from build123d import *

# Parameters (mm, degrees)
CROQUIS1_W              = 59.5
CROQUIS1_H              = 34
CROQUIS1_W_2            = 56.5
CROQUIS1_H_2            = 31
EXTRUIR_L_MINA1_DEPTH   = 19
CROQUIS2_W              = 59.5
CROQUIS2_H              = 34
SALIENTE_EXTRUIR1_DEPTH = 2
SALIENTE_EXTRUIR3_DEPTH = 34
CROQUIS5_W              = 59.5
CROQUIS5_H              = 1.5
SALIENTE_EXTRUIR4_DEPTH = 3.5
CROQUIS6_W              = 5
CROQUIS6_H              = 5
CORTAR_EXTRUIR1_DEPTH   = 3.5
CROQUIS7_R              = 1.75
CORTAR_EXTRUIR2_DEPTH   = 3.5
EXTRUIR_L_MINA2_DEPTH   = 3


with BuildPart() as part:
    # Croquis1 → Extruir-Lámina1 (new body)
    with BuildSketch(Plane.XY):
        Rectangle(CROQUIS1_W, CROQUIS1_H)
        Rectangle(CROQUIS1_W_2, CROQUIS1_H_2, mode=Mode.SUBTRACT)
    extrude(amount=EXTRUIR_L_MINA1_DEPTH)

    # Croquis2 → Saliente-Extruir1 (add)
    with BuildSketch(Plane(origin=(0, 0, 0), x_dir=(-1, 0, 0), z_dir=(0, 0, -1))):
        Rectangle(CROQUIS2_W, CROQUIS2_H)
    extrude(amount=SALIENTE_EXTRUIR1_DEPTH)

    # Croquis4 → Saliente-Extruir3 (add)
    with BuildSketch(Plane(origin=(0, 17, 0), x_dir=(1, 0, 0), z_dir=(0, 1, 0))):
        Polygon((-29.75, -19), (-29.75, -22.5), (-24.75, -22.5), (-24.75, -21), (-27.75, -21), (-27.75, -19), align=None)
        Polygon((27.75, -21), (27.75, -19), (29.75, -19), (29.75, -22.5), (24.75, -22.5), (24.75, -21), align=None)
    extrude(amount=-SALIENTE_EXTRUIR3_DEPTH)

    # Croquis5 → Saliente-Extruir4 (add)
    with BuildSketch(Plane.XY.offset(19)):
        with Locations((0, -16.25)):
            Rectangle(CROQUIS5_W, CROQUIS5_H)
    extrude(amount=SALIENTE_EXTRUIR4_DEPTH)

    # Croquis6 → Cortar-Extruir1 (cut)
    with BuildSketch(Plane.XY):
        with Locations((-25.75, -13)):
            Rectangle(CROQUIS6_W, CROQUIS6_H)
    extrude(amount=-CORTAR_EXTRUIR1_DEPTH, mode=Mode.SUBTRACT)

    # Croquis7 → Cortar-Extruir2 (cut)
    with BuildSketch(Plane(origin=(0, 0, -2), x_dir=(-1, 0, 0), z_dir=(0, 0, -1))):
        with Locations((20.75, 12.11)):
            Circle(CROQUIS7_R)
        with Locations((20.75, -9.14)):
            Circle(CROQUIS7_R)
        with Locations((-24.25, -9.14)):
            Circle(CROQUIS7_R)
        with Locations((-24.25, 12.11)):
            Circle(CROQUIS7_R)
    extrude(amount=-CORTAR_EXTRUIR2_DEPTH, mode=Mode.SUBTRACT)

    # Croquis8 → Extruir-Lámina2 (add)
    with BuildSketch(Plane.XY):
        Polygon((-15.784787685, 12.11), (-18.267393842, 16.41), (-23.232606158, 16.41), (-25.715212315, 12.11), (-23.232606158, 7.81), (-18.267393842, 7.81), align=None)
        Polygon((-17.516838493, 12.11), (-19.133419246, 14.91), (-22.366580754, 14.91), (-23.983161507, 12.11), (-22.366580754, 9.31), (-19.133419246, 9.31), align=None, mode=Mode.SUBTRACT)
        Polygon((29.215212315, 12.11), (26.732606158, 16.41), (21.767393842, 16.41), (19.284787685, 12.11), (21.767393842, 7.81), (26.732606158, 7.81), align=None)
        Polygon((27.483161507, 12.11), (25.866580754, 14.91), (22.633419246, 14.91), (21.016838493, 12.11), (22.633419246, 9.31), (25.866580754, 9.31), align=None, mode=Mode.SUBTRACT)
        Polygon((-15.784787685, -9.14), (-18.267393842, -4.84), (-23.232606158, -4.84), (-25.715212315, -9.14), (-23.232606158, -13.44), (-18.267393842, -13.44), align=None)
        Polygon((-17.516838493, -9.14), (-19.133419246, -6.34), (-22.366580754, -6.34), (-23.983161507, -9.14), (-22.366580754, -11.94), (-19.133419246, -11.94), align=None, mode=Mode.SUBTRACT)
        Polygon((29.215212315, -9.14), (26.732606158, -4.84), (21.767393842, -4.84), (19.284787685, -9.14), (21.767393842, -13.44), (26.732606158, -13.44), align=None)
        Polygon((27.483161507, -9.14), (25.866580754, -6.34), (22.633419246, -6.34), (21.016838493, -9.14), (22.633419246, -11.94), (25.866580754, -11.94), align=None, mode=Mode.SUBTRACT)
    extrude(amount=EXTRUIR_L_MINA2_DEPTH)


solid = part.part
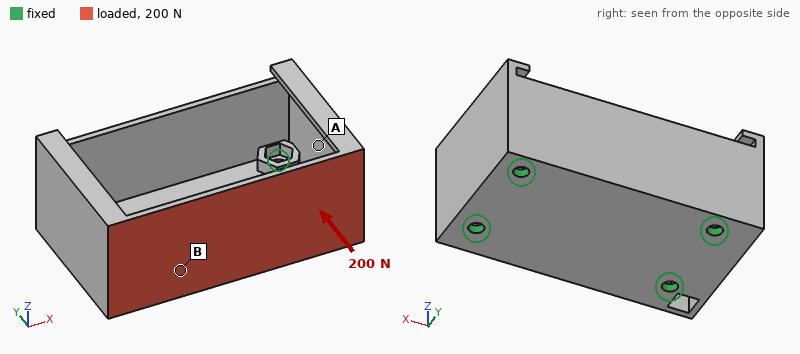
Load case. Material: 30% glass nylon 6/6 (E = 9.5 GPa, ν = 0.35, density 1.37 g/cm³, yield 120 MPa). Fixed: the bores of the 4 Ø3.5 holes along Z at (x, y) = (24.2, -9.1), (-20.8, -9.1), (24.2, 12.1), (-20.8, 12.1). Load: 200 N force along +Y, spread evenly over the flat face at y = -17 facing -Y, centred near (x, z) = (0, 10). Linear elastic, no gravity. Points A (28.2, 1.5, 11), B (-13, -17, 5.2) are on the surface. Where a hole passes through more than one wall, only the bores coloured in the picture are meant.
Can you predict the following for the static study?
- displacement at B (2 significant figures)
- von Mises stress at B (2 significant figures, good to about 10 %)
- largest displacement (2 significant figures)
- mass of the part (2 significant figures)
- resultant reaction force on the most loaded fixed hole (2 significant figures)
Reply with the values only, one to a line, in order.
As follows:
0.13 mm
15 MPa
0.82 mm
14 g
72 N
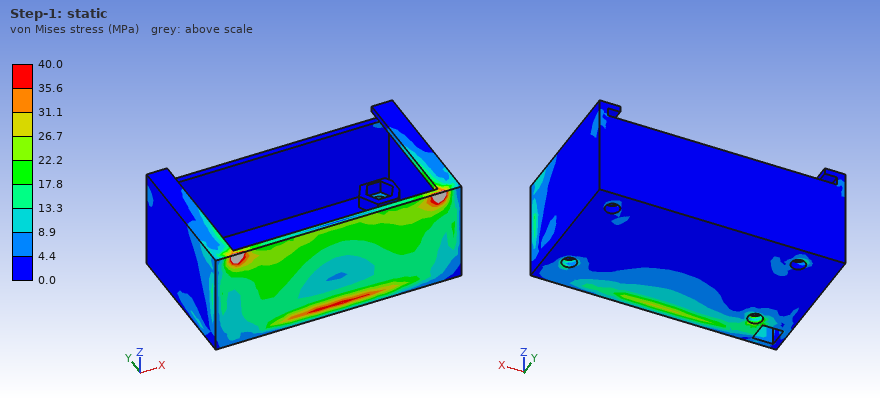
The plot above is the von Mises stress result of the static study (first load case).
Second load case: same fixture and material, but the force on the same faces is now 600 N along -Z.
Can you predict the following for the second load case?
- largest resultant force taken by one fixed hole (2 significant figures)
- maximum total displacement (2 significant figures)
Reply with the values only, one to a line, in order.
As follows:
390 N
0.42 mm
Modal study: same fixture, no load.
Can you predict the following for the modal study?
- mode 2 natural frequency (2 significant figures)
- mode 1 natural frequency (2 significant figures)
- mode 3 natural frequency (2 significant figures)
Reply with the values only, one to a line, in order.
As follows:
2200 Hz
2000 Hz
3600 Hz
